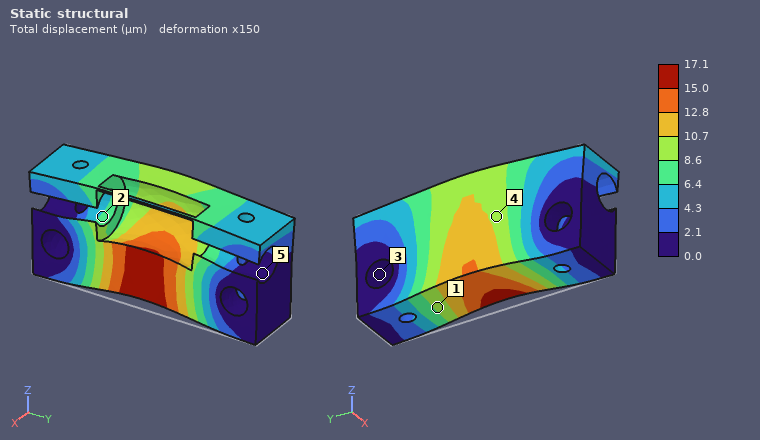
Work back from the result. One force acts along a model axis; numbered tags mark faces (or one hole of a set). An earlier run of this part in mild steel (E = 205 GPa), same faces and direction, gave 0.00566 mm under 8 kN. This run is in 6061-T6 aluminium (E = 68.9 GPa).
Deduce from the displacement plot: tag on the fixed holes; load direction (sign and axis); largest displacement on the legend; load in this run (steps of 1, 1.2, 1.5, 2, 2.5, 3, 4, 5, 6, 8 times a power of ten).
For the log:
3
+Z
17.1 µm
8 kN
